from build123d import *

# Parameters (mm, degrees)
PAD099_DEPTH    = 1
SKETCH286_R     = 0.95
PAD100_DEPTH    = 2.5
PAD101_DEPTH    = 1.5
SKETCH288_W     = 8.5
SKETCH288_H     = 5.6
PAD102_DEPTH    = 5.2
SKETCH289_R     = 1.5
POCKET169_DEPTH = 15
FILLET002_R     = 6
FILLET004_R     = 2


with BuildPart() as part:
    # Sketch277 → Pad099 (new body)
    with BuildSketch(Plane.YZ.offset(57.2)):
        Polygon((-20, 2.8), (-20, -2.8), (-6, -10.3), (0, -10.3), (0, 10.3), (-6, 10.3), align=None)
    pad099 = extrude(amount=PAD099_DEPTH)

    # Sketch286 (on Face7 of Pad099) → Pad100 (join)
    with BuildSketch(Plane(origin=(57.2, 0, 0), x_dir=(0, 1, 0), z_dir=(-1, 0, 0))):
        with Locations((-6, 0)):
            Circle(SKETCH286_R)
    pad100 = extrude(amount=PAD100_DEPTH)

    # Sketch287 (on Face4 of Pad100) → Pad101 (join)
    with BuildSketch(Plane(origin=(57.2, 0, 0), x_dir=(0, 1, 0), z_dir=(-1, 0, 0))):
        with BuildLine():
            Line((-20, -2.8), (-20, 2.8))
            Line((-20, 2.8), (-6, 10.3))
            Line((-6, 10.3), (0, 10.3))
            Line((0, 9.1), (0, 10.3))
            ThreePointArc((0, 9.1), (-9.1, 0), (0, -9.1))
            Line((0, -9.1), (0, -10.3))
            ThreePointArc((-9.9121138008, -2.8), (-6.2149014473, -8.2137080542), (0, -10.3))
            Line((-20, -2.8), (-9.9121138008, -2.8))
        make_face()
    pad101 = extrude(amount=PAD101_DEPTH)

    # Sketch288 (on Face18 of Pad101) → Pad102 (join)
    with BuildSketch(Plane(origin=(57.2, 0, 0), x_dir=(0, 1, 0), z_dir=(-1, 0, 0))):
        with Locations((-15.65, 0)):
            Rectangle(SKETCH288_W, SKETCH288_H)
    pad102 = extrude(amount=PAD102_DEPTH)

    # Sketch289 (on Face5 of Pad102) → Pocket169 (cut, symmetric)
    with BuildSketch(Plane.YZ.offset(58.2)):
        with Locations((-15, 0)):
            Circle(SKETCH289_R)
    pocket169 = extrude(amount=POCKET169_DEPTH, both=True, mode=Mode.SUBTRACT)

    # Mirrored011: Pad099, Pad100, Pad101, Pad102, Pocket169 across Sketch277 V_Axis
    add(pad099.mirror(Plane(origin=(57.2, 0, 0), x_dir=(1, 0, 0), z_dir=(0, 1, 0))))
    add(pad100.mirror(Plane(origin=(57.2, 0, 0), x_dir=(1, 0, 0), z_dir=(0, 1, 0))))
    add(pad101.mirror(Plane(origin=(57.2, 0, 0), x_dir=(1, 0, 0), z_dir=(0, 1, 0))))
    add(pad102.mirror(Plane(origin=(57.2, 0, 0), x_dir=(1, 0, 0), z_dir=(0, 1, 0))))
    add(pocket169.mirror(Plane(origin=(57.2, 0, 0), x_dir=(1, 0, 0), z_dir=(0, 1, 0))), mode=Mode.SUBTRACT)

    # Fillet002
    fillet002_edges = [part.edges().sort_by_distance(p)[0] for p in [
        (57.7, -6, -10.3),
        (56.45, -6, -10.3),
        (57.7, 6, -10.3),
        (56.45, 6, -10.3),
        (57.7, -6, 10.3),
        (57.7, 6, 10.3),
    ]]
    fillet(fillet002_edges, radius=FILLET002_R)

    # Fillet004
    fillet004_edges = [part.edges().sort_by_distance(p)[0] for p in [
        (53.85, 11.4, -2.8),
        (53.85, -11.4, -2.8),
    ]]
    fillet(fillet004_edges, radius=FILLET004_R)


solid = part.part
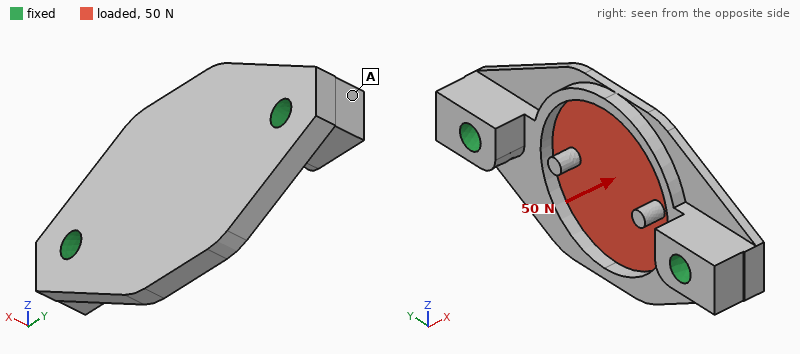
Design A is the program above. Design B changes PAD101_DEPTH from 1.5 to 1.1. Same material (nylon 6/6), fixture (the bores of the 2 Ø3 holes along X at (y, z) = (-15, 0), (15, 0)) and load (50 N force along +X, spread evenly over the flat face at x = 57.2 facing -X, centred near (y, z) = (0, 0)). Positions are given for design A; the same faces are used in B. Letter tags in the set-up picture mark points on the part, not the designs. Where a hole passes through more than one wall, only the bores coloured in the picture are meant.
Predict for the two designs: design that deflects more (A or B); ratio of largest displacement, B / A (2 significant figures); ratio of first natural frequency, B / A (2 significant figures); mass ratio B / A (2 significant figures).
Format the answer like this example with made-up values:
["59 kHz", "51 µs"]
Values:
["B", "1.4", "0.87", "0.95"]
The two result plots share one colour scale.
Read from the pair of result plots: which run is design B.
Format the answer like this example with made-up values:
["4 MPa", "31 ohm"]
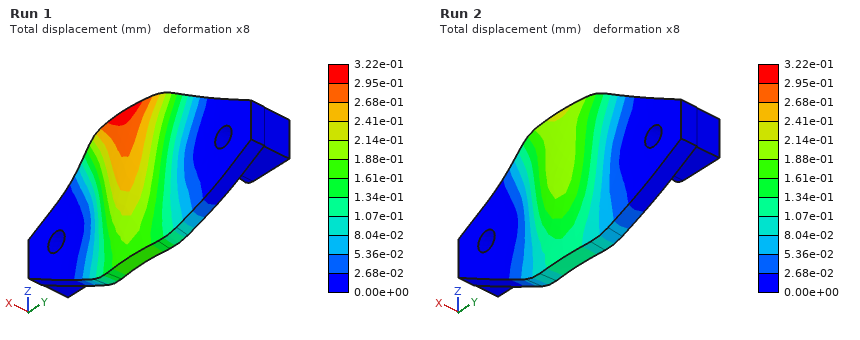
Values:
["Run 1"]
